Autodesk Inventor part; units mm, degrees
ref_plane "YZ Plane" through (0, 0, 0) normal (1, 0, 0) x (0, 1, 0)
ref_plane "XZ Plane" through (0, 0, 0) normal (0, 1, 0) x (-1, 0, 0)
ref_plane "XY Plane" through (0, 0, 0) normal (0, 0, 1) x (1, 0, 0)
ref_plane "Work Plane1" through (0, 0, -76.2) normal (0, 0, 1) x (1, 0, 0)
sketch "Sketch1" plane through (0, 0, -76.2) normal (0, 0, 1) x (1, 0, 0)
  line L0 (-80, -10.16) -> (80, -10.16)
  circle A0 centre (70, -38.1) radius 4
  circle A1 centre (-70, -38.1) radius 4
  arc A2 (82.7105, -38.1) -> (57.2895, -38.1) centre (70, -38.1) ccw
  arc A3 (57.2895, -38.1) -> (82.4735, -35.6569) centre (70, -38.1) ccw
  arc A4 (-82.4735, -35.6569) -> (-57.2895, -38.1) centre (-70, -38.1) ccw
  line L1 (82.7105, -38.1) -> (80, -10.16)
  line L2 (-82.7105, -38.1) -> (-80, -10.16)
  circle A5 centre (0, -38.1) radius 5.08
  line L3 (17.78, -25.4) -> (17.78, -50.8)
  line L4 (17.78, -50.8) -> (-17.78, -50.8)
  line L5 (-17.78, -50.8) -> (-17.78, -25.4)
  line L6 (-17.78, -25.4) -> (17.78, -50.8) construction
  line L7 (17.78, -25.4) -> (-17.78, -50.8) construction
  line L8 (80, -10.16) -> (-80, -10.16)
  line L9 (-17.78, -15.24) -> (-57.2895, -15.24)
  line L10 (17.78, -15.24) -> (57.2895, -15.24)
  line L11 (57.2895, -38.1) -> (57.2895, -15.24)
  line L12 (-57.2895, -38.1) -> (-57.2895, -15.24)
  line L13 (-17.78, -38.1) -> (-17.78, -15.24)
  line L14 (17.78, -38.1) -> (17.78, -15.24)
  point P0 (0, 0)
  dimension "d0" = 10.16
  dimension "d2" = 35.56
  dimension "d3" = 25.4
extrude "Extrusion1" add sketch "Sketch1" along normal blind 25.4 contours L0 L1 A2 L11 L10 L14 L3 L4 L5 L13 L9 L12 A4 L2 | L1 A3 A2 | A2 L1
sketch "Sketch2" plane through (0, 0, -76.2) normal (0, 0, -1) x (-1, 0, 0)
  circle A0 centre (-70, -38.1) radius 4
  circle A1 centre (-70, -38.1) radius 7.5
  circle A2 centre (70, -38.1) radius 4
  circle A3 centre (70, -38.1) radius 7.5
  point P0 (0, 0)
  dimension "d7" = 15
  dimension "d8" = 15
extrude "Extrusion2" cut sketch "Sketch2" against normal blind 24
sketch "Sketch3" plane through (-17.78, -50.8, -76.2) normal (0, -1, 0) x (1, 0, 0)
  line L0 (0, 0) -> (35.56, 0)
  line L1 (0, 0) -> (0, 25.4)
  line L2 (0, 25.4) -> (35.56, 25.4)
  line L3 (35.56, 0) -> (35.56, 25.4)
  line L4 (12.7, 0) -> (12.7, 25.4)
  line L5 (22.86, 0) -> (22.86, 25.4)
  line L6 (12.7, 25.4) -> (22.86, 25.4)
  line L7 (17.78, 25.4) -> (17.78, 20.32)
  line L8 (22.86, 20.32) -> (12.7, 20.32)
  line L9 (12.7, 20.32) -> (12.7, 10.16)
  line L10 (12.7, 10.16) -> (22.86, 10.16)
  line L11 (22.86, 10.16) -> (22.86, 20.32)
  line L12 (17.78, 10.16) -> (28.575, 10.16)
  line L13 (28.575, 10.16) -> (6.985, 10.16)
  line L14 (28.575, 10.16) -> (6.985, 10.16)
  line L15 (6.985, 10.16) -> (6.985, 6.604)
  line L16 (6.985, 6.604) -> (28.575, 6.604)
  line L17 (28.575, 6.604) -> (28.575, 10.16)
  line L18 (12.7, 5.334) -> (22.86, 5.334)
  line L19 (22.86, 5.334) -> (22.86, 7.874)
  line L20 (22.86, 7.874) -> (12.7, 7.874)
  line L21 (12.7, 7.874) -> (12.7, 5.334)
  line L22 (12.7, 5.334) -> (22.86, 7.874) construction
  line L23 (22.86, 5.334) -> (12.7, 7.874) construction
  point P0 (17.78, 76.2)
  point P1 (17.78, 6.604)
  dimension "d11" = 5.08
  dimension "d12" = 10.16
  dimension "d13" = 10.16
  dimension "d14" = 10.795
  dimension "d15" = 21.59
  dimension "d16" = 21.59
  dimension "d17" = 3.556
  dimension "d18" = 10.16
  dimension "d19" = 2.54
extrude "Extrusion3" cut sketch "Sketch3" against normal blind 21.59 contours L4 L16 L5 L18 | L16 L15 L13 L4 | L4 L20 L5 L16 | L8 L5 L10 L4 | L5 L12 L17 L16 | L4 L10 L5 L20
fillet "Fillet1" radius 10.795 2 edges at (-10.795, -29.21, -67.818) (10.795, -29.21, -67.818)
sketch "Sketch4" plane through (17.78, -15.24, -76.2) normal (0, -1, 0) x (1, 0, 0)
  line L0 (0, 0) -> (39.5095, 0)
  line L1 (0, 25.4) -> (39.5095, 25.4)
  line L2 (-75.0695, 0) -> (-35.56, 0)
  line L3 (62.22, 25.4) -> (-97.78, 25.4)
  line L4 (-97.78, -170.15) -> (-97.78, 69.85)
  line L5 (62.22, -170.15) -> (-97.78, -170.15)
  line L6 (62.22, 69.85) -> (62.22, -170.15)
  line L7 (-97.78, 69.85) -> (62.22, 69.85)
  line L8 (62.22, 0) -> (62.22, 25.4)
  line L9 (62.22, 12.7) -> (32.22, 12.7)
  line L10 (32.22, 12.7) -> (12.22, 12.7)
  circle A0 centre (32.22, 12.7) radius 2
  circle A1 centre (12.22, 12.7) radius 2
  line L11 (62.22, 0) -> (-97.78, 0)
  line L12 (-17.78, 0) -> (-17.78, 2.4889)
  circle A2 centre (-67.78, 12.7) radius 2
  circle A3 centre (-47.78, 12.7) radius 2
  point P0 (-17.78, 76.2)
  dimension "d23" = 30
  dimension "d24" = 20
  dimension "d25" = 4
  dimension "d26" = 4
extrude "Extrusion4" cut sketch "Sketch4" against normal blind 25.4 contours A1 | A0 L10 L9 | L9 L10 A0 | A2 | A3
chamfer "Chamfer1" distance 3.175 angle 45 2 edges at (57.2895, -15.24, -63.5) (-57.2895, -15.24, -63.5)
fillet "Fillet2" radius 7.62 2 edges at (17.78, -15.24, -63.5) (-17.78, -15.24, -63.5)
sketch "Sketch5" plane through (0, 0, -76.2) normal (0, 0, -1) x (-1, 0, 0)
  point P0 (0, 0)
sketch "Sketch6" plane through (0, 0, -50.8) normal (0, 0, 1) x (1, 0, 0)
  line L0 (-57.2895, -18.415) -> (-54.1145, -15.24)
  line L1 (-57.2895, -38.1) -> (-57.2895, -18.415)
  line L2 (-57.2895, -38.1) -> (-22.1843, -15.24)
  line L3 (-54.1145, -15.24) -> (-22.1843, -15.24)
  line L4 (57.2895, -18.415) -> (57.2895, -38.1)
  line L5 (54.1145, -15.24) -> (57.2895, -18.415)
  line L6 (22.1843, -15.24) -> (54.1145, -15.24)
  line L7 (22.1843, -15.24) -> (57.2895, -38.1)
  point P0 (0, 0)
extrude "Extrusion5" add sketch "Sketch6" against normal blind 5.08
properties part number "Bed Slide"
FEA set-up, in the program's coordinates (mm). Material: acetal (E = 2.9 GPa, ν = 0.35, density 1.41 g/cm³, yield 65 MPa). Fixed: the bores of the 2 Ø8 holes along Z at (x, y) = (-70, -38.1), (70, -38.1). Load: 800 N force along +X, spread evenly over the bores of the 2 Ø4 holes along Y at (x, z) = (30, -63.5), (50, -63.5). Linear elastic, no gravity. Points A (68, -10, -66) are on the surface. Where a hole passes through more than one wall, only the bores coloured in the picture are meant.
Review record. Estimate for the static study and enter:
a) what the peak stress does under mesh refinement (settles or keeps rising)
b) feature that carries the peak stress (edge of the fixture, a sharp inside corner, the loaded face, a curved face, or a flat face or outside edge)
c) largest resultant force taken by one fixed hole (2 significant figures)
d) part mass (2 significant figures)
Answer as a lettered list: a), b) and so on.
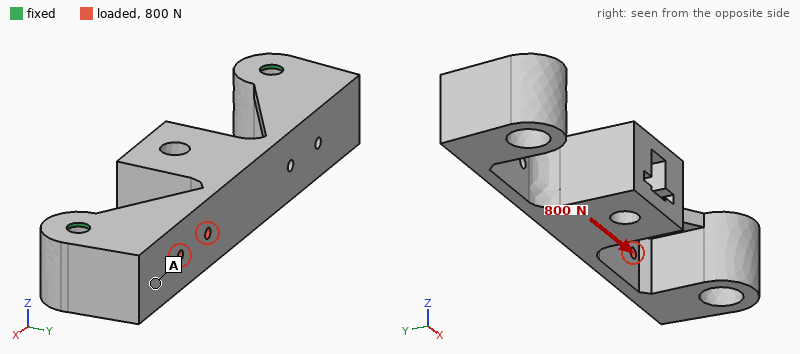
a) keeps rising
b) edge of the fixture
c) 420 N
d) 120 g
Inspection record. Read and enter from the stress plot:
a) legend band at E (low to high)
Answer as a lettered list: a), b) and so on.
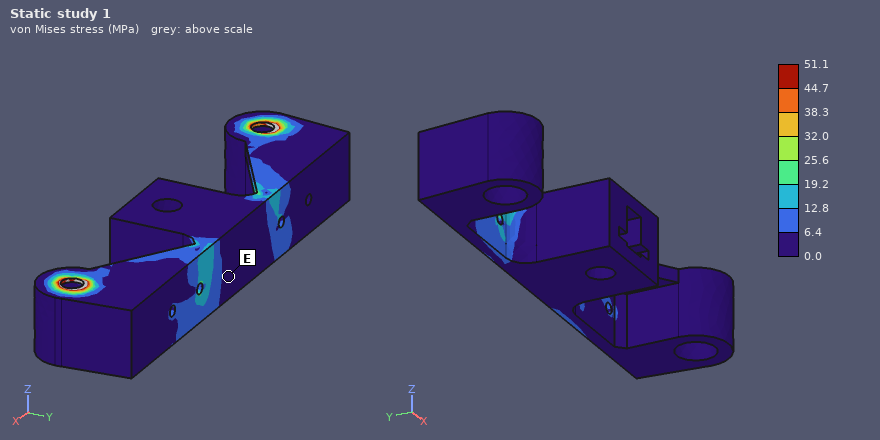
a) 0.0 to 6.4 MPa
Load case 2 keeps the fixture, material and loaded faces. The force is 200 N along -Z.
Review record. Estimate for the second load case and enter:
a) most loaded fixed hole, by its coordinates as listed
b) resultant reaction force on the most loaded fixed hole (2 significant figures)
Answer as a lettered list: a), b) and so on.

a) (70, -38.1)
b) 160 N
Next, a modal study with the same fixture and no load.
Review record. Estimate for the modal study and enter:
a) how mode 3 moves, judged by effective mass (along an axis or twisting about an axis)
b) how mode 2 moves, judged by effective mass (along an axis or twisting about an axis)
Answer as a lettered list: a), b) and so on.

a) along X
b) along Z
